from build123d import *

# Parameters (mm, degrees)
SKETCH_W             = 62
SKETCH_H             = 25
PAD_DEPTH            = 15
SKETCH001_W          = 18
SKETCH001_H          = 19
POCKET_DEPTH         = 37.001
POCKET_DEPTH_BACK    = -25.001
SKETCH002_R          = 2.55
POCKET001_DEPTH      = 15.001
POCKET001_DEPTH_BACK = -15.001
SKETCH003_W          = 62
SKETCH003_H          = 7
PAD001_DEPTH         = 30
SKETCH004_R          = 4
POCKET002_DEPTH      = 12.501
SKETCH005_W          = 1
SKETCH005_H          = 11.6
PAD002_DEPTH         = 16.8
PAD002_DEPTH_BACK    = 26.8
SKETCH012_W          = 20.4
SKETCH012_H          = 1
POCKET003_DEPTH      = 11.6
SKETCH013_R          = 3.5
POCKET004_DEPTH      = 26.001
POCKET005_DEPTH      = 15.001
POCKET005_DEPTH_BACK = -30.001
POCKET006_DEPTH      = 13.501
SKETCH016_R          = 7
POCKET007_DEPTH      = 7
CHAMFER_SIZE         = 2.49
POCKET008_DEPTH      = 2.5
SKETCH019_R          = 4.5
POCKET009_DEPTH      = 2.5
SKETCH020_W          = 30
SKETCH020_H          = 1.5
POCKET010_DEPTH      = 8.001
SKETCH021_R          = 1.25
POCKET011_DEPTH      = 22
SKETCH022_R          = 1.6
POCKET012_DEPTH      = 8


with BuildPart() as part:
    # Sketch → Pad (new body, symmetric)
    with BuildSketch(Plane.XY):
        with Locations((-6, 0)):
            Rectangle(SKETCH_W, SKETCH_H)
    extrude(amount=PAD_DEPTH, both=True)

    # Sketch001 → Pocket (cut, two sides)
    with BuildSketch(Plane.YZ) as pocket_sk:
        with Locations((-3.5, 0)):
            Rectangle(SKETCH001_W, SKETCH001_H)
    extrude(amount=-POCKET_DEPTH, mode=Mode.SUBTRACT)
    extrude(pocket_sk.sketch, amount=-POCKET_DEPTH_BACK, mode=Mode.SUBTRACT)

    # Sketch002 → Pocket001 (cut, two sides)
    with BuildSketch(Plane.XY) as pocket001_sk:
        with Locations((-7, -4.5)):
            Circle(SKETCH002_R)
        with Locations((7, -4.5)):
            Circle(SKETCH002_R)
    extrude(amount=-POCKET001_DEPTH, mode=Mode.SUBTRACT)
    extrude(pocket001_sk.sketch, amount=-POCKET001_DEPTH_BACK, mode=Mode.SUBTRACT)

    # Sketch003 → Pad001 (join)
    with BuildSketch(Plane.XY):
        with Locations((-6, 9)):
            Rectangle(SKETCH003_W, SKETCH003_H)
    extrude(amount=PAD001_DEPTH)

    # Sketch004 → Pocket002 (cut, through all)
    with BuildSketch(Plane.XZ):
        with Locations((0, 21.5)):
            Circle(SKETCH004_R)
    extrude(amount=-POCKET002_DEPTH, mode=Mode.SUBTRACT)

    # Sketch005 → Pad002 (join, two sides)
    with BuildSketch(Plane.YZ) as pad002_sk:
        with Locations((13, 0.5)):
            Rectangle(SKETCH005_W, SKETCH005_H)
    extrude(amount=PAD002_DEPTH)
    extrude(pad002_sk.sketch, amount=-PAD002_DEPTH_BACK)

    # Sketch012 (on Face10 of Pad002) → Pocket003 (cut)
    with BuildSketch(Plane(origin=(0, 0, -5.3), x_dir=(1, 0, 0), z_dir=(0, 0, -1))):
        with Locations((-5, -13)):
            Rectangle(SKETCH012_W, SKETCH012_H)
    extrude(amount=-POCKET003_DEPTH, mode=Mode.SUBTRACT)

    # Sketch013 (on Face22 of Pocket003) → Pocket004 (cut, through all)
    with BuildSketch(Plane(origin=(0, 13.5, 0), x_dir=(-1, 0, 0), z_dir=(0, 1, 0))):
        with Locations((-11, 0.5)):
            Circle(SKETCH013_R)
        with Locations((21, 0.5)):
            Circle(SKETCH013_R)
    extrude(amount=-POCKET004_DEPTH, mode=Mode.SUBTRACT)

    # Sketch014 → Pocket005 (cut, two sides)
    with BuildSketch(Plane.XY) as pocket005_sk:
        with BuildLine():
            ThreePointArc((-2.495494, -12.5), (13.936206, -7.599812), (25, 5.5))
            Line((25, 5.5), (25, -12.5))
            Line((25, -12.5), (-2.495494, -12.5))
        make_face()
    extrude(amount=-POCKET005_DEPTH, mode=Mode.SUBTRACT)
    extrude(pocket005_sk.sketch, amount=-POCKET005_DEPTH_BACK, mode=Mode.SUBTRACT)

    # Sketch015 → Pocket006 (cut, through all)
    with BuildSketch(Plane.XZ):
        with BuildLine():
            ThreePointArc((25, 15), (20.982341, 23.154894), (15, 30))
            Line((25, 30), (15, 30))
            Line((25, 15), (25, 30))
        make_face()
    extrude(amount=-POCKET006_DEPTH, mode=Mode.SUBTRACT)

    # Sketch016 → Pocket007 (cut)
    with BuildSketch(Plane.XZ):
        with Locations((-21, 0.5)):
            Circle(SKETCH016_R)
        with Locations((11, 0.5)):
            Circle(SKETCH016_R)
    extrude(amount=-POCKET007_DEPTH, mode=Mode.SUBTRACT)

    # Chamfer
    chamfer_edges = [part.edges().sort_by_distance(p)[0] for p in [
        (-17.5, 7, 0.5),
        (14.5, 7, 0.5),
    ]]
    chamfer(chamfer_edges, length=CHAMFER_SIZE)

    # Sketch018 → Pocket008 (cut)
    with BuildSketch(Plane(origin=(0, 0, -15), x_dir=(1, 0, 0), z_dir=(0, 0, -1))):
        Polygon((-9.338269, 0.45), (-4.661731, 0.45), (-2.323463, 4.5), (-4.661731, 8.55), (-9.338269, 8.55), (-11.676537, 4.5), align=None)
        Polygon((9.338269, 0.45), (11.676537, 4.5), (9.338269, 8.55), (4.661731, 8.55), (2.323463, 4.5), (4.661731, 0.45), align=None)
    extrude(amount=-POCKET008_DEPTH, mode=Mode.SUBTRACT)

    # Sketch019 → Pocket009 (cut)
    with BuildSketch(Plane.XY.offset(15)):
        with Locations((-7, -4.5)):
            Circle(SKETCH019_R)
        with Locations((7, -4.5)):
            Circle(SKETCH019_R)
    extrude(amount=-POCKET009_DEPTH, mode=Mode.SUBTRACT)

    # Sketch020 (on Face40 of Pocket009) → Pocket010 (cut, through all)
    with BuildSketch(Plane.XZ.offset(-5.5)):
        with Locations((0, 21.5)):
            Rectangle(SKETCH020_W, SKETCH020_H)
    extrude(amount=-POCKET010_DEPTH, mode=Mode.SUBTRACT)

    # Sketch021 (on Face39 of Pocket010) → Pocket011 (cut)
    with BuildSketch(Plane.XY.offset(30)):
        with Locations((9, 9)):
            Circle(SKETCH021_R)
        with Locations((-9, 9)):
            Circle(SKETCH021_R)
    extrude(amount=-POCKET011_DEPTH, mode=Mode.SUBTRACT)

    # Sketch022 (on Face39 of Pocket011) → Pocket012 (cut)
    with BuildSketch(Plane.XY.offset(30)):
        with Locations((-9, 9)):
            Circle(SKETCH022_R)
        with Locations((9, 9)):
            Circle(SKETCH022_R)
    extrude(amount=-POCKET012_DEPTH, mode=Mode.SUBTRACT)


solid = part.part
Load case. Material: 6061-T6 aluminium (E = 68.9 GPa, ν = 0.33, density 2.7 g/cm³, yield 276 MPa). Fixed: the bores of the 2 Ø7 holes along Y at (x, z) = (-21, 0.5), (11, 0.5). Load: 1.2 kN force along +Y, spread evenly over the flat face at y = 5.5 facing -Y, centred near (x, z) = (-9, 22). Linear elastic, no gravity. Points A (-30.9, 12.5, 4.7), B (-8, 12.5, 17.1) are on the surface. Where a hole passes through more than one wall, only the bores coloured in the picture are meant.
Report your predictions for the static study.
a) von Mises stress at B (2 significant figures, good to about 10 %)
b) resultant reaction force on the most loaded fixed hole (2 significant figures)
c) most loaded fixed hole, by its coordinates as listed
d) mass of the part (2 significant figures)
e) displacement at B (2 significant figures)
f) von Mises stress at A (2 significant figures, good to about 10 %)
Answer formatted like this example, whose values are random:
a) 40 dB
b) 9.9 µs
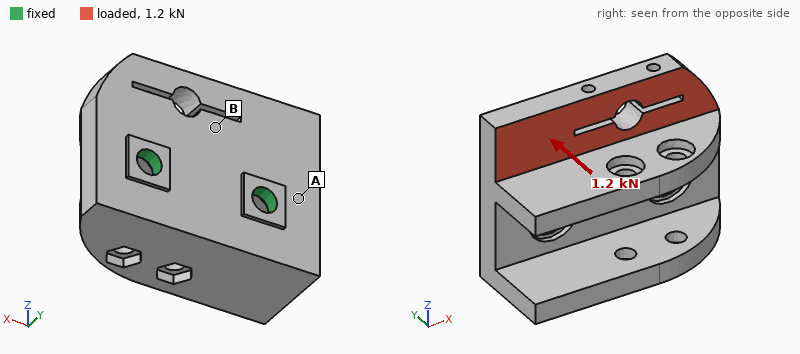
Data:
a) 14 MPa
b) 730 N
c) (-21, 0.5)
d) 74 g
e) 0.041 mm
f) 34 MPa
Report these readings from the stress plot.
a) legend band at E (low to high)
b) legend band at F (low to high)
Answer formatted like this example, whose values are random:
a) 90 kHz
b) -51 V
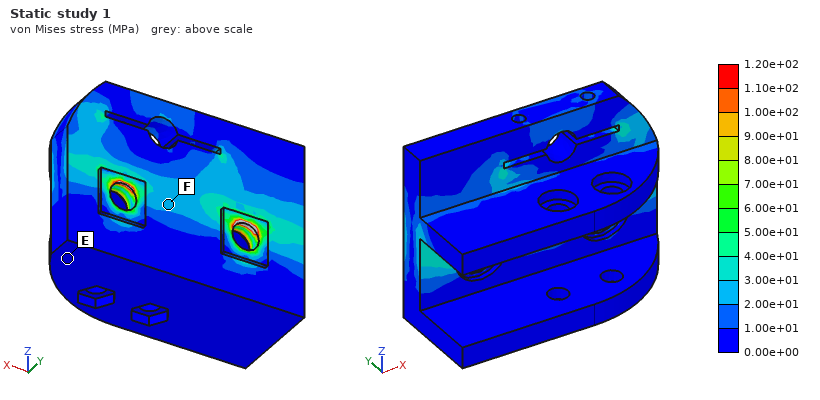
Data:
a) 0.00e+00 to 1.00e+01 MPa
b) 2.00e+01 to 3.00e+01 MPa
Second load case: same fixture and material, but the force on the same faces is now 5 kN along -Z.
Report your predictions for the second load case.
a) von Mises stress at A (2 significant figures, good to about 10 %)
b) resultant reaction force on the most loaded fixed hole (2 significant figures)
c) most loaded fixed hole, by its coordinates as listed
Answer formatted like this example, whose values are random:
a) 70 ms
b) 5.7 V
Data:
a) 28 MPa
b) 3.0 kN
c) (-21, 0.5)
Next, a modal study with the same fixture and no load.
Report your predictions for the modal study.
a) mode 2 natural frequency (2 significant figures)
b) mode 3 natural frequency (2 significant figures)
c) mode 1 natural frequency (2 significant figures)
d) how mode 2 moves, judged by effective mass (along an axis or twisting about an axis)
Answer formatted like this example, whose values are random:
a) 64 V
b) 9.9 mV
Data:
a) 6500 Hz
b) 7100 Hz
c) 3900 Hz
d) along Y
